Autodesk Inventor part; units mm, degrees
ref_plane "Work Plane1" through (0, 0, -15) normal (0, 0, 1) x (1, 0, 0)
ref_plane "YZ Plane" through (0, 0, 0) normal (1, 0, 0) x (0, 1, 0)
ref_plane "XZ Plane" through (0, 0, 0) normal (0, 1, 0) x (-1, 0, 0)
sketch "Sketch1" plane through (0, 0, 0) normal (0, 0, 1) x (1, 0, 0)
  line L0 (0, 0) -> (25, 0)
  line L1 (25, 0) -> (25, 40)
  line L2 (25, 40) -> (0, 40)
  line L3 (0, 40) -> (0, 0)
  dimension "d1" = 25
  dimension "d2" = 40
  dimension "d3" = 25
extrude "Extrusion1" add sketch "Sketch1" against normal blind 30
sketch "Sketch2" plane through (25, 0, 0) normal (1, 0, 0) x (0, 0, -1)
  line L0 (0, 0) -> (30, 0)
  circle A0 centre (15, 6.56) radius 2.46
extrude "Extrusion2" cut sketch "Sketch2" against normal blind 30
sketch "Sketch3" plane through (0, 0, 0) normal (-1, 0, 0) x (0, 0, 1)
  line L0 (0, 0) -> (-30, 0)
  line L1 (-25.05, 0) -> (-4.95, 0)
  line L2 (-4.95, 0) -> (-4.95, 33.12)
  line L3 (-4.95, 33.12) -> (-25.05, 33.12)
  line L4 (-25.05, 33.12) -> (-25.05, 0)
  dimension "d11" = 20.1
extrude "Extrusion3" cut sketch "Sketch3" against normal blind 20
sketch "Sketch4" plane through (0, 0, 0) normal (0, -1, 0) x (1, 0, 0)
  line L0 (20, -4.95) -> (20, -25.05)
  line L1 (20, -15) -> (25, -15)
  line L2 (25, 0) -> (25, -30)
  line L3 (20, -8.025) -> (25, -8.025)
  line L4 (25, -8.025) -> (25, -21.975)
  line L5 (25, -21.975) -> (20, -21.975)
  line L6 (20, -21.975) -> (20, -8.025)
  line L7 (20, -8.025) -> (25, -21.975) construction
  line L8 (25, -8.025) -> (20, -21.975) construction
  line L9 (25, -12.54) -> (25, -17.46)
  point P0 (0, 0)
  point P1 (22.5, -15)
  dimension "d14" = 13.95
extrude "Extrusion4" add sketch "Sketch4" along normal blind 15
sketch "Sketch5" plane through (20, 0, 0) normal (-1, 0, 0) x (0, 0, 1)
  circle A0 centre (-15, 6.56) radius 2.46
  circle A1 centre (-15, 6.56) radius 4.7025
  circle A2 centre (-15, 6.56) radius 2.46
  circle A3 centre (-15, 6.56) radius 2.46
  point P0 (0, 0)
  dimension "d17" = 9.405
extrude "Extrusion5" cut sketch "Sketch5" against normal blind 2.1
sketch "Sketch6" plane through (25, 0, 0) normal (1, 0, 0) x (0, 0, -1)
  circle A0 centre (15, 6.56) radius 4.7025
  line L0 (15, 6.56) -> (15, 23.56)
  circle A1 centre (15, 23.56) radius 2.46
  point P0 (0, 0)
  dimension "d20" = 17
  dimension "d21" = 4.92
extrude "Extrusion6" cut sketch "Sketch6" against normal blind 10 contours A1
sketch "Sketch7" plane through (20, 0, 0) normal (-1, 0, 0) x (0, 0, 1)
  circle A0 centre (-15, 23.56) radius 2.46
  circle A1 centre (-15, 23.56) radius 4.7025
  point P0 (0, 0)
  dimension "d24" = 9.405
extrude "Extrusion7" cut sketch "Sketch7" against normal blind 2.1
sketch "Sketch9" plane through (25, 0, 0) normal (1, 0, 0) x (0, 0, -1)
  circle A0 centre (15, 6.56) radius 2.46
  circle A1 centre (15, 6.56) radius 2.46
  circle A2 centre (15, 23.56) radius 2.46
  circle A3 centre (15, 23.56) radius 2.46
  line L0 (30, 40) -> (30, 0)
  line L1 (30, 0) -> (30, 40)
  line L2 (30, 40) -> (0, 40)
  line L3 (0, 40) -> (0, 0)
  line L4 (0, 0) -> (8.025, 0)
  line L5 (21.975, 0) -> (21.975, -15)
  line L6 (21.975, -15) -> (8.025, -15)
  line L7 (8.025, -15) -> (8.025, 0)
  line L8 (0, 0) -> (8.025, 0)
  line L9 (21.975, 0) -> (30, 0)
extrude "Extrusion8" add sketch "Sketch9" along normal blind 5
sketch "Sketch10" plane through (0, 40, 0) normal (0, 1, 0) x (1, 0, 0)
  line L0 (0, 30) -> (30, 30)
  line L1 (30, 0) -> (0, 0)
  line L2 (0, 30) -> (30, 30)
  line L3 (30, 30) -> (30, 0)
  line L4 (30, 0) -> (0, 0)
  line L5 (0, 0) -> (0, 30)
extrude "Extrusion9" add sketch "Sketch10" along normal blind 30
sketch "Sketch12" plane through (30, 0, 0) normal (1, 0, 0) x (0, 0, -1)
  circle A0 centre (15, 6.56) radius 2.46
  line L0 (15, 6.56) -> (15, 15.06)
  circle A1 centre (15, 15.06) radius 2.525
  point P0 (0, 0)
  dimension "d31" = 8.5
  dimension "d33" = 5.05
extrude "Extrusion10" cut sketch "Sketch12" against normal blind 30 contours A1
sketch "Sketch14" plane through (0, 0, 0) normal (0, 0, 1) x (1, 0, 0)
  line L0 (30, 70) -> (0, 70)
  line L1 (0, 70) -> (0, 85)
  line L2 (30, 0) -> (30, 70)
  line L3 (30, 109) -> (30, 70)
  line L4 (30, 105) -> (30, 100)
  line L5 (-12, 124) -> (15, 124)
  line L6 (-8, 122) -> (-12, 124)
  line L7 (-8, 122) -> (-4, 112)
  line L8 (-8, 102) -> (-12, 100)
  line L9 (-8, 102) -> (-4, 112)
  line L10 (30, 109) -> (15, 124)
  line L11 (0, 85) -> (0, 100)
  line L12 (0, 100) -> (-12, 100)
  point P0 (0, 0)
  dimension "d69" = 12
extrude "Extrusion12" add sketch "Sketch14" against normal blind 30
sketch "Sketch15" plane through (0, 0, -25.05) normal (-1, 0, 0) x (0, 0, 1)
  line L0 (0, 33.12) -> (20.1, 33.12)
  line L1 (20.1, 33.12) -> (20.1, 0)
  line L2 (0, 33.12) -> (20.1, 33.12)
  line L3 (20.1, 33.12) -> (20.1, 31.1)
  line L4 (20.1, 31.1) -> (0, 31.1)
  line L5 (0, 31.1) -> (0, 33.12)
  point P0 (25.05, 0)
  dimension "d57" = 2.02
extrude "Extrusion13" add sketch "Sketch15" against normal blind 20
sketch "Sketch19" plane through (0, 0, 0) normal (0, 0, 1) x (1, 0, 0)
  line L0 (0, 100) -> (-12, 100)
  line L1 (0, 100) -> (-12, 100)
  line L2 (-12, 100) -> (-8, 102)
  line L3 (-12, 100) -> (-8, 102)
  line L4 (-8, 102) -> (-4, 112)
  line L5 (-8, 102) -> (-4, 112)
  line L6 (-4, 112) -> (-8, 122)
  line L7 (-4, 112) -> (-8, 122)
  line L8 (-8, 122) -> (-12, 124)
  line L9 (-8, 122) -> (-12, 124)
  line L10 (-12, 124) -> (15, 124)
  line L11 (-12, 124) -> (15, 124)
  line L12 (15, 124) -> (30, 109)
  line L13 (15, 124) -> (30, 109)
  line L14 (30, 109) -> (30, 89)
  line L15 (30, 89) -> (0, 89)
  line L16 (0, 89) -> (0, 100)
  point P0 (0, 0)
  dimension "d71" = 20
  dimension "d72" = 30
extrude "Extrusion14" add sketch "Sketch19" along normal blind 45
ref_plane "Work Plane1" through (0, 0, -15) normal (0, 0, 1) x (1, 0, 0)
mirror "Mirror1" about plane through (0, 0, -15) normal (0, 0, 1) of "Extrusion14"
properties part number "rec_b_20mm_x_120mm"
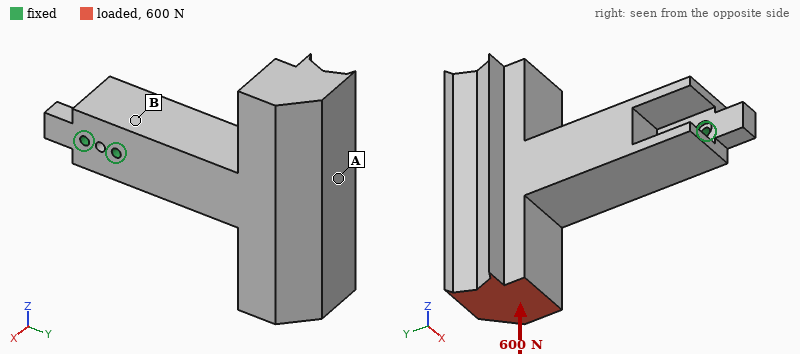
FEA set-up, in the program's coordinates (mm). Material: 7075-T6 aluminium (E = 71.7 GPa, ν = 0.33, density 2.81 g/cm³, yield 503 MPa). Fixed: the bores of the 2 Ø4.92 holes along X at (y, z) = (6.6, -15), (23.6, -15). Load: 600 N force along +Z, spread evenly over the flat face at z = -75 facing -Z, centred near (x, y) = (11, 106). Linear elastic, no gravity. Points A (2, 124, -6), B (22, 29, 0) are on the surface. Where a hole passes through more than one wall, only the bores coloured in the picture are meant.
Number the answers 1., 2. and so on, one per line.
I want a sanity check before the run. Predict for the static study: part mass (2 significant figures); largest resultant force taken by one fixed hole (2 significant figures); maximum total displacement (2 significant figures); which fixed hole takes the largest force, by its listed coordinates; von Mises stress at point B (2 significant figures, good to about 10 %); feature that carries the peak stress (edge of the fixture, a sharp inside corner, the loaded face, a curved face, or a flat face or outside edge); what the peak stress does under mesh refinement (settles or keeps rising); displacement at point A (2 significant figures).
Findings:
1. 560 g
2. 2.7 kN
3. 0.12 mm
4. (23.6, -15)
5. 20 MPa
6. edge of the fixture
7. keeps rising
8. 0.10 mm
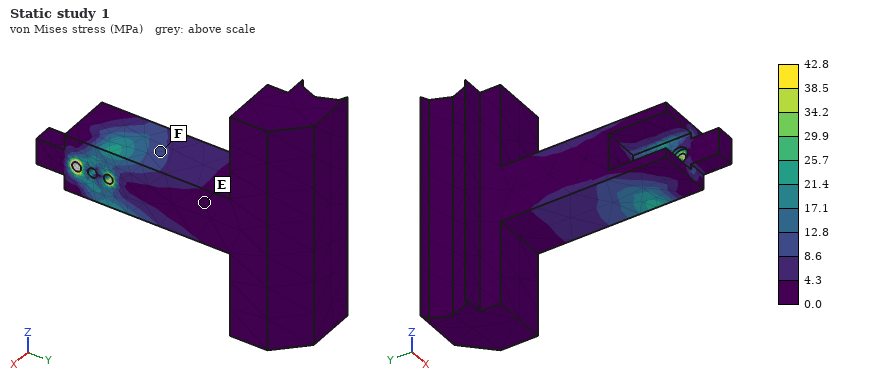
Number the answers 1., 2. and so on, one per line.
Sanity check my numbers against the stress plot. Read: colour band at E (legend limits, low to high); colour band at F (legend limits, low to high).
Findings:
1. 0.0 to 4.3 MPa
2. 8.6 to 12.8 MPa
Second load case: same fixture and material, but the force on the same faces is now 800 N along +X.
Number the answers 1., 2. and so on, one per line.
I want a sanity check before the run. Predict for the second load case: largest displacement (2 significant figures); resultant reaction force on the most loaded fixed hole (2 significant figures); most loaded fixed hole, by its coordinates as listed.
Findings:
1. 0.39 mm
2. 3.4 kN
3. (23.6, -15)
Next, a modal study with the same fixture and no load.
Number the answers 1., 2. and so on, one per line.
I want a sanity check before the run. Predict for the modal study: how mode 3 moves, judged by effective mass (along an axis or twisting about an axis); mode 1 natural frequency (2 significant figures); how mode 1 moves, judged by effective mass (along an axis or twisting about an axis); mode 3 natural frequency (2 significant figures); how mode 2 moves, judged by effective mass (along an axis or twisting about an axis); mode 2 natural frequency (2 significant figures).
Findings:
1. twisting about Y
2. 580 Hz
3. along X
4. 880 Hz
5. along Z
6. 620 Hz
